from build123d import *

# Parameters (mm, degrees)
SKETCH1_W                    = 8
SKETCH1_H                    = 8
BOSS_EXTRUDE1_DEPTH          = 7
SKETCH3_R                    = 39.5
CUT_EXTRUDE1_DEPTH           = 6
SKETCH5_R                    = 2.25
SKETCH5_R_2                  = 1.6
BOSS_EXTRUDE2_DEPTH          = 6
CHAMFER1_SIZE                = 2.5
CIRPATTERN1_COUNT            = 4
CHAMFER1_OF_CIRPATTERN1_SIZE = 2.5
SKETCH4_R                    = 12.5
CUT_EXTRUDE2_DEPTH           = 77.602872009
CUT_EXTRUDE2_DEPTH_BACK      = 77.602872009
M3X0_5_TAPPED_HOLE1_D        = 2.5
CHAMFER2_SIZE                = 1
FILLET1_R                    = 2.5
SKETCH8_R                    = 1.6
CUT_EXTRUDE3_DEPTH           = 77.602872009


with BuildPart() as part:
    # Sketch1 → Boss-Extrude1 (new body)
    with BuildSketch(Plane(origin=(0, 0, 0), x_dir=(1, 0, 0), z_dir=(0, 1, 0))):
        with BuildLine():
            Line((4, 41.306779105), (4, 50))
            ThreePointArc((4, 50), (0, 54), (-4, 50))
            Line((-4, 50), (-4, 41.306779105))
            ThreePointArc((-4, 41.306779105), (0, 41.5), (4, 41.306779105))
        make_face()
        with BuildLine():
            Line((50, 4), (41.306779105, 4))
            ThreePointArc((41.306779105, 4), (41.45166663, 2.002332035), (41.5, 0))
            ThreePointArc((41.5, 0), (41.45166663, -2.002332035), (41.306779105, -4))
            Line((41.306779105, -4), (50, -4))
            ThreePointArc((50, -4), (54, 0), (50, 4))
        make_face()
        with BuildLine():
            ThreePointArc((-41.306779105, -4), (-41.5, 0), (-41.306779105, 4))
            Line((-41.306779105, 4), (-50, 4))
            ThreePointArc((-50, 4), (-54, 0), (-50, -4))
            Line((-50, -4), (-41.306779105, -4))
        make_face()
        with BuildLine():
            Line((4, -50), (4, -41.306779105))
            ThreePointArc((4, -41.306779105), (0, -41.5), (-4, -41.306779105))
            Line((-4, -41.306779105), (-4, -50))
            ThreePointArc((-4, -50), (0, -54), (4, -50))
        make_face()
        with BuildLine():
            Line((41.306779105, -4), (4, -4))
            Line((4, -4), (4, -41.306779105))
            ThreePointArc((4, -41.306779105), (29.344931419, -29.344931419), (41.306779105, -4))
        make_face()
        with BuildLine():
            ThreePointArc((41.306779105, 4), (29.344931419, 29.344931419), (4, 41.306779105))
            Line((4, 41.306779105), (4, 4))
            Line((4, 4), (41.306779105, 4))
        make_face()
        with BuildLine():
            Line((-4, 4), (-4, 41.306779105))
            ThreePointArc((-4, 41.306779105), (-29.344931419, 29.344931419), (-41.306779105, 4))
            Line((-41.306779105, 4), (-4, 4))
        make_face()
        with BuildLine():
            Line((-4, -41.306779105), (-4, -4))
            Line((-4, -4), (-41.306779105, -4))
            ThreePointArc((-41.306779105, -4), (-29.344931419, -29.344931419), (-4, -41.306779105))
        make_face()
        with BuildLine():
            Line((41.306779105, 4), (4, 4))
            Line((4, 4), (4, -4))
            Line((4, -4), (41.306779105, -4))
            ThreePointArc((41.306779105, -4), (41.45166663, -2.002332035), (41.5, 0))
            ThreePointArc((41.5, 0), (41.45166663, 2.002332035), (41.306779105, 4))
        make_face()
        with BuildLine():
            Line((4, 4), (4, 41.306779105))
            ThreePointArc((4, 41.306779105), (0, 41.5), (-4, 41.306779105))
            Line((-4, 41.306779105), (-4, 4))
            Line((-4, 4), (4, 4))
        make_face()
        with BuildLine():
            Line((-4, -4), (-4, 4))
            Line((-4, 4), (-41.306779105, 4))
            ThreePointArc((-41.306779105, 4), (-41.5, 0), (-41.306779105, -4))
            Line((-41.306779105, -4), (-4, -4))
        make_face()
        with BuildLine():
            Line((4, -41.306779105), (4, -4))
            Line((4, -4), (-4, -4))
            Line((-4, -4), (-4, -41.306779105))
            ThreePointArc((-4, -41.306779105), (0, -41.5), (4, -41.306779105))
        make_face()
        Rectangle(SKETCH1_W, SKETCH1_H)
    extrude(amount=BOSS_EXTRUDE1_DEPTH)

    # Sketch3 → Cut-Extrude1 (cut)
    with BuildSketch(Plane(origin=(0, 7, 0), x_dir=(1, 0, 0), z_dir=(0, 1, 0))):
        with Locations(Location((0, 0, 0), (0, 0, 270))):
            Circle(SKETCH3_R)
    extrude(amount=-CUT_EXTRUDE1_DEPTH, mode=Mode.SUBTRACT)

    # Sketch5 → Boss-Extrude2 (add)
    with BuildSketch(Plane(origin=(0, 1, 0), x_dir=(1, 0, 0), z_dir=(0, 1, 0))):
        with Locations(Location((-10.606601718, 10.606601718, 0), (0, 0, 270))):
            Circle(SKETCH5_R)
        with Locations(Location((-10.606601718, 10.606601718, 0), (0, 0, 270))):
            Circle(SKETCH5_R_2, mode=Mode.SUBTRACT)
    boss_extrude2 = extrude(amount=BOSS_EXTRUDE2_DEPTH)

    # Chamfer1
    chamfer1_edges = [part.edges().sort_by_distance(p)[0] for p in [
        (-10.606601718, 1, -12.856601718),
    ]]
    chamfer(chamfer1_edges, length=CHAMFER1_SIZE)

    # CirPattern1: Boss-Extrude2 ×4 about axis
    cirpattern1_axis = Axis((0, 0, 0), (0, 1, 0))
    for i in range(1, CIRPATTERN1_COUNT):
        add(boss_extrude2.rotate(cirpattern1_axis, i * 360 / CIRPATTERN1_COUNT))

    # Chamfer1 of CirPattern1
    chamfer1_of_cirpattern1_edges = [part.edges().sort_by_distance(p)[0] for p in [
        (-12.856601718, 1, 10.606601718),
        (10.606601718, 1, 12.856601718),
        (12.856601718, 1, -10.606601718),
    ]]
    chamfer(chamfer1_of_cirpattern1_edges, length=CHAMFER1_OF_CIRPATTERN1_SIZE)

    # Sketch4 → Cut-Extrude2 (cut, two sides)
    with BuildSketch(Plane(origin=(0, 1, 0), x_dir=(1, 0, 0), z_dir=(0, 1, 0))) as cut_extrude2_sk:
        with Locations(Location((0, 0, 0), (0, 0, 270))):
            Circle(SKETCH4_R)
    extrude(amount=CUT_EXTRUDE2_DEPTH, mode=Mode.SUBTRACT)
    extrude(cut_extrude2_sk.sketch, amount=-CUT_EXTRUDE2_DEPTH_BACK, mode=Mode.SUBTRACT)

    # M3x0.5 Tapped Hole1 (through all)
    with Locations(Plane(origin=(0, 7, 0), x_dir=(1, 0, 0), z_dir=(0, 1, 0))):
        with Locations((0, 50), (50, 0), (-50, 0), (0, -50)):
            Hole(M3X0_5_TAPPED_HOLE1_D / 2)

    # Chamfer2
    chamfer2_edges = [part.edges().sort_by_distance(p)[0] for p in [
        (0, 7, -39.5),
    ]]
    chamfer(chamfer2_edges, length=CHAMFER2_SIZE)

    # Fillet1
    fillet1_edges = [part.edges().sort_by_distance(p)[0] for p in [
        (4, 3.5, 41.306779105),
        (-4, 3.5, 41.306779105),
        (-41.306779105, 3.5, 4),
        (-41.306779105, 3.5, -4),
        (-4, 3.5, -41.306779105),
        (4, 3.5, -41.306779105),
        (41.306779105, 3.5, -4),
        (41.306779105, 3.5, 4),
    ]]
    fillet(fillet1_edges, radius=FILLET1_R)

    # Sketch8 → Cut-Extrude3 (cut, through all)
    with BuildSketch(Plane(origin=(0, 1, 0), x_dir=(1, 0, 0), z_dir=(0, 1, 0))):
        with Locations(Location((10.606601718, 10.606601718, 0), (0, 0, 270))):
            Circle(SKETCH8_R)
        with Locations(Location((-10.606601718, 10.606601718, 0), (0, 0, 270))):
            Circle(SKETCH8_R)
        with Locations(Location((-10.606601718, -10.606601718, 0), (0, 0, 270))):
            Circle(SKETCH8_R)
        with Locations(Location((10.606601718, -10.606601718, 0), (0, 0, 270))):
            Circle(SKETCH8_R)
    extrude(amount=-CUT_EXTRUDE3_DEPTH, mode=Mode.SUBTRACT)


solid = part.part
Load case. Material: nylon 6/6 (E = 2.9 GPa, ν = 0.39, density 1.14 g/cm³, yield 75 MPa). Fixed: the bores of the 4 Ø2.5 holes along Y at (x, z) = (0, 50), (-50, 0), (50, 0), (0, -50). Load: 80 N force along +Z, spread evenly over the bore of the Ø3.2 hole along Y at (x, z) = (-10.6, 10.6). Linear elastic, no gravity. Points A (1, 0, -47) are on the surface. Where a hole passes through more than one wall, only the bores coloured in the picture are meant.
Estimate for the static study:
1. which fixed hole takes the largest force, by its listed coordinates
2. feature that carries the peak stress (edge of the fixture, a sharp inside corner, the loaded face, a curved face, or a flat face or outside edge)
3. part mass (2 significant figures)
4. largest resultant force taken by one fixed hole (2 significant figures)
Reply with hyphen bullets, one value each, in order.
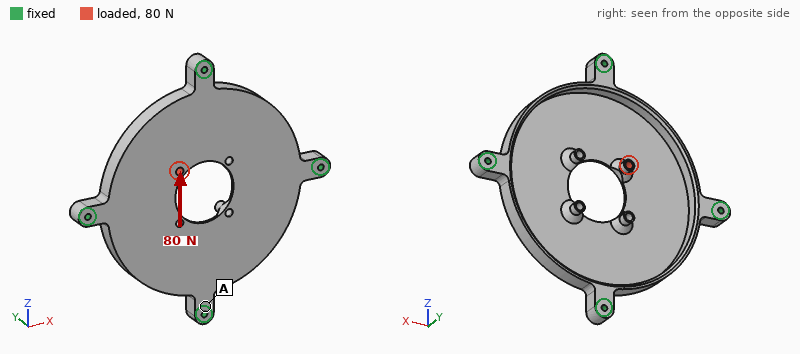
- (0, 50)
- a curved face
- 12 g
- 35 N
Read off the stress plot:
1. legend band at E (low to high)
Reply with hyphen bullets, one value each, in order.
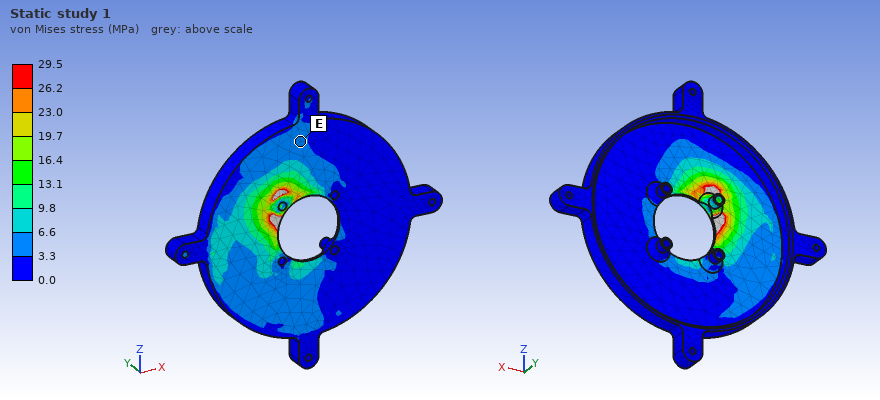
- 3.3 to 6.6 MPa
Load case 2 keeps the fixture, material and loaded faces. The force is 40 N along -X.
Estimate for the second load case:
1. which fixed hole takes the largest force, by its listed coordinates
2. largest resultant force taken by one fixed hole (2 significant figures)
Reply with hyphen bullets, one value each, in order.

- (-50, 0)
- 18 N
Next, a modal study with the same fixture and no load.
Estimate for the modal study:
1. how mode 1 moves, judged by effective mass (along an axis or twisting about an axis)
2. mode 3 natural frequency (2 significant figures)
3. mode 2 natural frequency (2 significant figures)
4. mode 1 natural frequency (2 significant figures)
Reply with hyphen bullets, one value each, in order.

- along Y
- 910 Hz
- 900 Hz
- 500 Hz
